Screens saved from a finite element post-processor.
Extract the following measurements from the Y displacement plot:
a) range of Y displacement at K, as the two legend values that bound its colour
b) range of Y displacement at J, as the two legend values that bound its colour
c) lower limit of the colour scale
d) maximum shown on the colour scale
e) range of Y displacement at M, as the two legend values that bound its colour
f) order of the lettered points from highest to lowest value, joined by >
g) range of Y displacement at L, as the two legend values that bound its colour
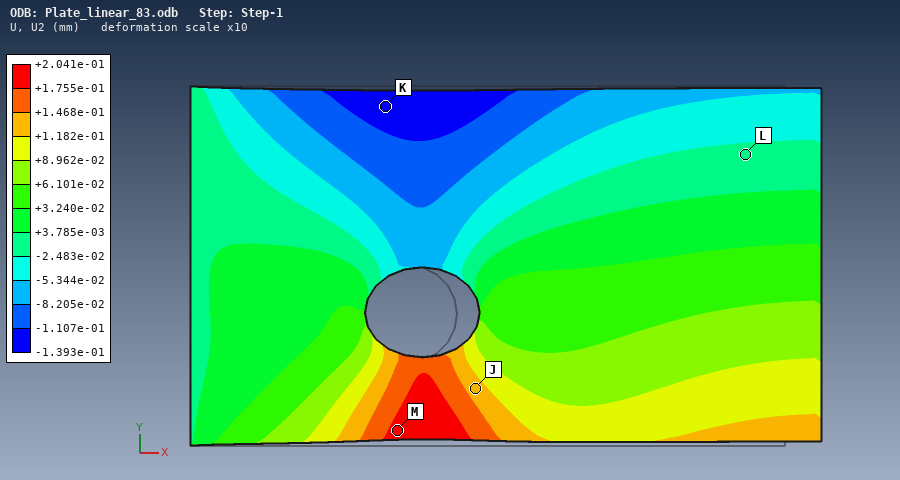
-1.393e-01 to -1.107e-01 mm
+1.182e-01 to +1.468e-01 mm
-1.393e-01 mm
+2.041e-01 mm
+1.755e-01 to +2.041e-01 mm
M > J > L > K
-2.483e-02 to +3.785e-03 mm
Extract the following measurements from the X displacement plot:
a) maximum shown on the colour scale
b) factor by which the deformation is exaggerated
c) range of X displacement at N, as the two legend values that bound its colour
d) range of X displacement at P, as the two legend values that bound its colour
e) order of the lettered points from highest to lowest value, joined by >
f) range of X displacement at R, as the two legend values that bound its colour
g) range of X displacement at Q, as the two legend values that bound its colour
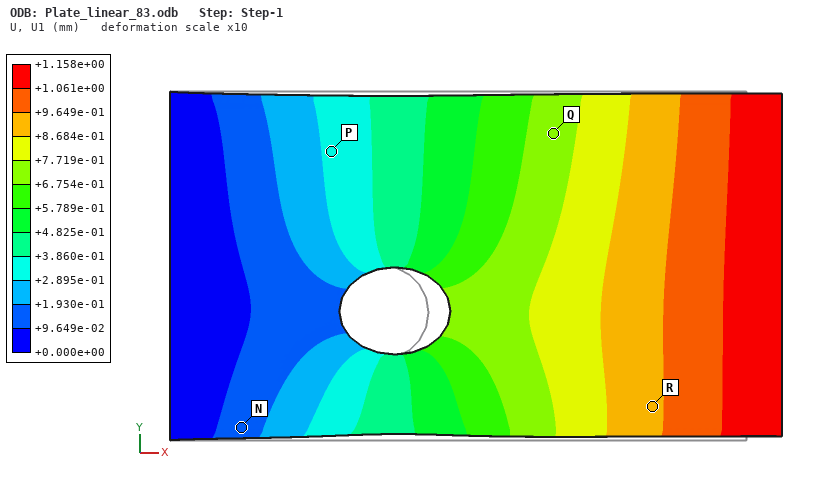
+1.158e+00 mm
10
+9.649e-02 to +1.930e-01 mm
+2.895e-01 to +3.860e-01 mm
R > Q > P > N
+8.684e-01 to +9.649e-01 mm
+6.754e-01 to +7.719e-01 mm
